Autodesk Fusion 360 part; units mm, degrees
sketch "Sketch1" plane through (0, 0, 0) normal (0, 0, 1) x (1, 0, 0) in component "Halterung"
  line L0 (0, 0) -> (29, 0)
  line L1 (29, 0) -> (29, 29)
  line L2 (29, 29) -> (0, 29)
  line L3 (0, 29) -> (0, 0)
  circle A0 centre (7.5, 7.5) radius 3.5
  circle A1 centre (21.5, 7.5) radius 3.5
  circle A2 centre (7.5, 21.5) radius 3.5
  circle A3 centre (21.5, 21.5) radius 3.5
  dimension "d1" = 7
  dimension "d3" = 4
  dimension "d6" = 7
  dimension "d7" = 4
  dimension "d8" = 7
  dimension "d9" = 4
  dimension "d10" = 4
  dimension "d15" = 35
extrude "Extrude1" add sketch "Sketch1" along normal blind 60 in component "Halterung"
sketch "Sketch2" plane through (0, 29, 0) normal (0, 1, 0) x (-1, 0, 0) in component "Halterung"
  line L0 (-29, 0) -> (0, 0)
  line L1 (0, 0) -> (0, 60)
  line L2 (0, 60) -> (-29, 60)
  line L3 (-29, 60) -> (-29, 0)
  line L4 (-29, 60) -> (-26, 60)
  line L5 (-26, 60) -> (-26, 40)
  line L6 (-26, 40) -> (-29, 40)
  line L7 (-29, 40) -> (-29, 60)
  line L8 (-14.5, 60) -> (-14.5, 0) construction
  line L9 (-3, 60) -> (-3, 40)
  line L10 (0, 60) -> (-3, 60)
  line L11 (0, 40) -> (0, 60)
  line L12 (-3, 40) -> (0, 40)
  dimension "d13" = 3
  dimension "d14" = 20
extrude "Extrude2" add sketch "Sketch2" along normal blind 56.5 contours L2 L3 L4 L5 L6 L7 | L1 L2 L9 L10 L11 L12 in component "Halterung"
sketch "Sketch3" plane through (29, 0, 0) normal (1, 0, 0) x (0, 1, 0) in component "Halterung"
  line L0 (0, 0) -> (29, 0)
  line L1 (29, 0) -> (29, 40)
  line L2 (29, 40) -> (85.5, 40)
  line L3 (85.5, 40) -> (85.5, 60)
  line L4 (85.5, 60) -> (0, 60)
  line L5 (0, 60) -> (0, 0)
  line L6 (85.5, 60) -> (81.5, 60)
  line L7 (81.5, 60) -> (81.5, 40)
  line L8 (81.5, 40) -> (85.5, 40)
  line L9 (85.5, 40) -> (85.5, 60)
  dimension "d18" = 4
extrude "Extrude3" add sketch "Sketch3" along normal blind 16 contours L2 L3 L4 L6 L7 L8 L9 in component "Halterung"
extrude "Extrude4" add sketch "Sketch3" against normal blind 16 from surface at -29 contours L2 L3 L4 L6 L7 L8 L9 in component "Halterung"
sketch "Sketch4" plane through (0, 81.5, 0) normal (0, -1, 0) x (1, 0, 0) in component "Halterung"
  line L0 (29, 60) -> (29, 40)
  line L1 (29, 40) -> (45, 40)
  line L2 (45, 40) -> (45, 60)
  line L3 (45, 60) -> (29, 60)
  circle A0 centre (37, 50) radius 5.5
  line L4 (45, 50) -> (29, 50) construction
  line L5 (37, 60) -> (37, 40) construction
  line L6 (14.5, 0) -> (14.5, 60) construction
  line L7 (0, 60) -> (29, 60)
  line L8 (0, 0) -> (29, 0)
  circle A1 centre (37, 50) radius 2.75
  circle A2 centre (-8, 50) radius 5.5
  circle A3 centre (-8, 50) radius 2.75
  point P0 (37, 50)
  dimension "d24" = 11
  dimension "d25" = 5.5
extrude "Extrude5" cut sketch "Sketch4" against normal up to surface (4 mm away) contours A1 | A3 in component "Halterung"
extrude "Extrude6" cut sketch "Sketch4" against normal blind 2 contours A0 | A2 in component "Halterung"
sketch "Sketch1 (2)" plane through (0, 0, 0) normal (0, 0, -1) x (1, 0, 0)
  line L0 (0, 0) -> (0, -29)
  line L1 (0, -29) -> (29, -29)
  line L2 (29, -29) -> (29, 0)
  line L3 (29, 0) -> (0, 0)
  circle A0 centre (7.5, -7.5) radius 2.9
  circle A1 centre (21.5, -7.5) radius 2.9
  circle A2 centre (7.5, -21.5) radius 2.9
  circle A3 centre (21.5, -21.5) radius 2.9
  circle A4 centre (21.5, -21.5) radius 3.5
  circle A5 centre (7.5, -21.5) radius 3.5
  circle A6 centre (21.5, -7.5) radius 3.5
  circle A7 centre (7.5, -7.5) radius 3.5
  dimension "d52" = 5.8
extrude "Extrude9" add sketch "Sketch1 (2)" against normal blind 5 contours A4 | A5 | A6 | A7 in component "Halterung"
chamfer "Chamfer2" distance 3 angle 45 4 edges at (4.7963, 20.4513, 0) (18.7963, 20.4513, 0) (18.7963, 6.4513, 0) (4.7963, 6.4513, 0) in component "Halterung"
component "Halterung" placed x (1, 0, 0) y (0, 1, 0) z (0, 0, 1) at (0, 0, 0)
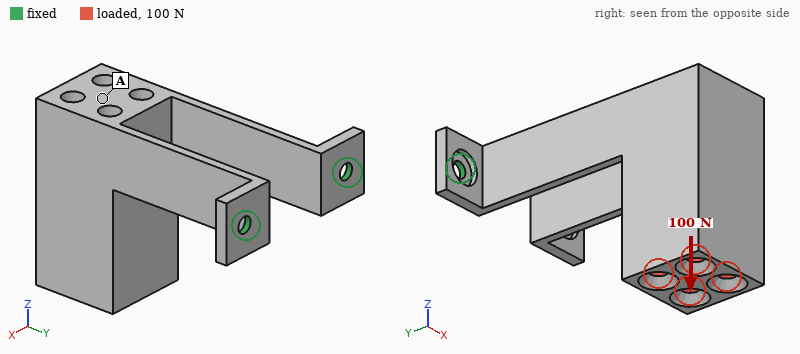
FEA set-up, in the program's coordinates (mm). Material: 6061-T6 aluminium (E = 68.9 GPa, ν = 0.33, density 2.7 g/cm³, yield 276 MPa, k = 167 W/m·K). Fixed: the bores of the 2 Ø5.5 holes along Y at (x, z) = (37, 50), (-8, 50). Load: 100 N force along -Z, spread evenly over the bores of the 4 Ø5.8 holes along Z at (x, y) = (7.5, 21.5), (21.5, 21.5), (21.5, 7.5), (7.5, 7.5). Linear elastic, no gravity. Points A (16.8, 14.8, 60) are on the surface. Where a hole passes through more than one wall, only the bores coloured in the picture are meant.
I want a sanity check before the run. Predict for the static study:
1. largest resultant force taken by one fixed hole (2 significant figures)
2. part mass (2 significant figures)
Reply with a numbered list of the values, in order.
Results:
1. 50 N
2. 130 g
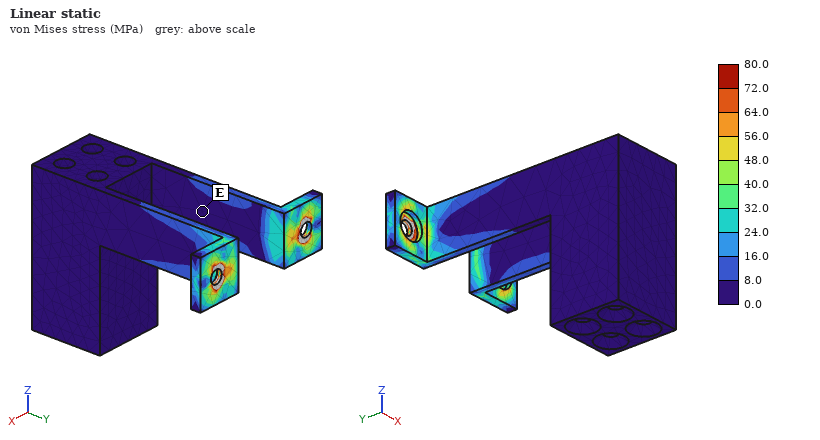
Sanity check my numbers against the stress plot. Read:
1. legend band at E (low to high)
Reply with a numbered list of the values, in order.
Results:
1. 0.0 to 8.0 MPa
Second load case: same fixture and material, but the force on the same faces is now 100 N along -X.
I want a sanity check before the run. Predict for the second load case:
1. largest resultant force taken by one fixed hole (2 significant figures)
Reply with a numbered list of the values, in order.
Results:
1. 220 N
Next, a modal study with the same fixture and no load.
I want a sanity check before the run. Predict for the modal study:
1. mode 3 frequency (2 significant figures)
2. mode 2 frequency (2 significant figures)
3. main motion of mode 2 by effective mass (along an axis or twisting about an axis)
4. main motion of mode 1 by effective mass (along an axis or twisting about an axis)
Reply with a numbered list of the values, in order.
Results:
1. 740 Hz
2. 270 Hz
3. along X
4. along Z
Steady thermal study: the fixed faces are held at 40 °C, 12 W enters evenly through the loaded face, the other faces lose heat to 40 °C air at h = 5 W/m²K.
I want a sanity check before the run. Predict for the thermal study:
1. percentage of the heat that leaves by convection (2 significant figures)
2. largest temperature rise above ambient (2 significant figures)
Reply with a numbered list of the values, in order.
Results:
1. 22 %
2. 37 K
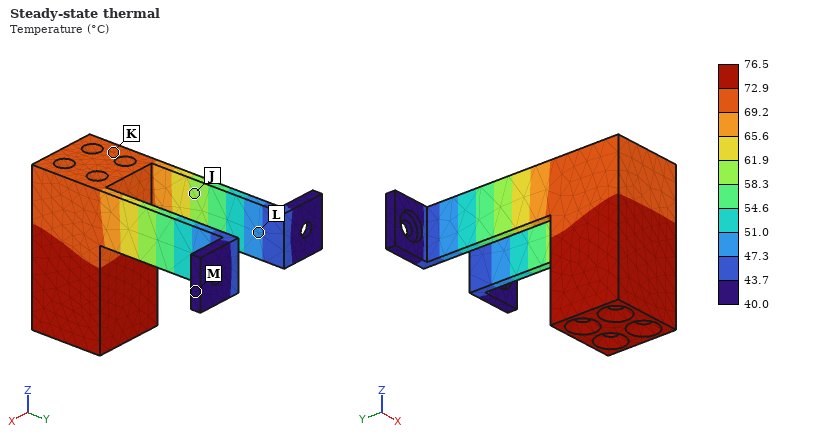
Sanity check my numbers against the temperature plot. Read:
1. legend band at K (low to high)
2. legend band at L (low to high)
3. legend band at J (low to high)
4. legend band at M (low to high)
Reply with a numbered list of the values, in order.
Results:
1. 69.2 to 72.9 °C
2. 47.3 to 51.0 °C
3. 58.3 to 61.9 °C
4. 40.0 to 43.7 °C
